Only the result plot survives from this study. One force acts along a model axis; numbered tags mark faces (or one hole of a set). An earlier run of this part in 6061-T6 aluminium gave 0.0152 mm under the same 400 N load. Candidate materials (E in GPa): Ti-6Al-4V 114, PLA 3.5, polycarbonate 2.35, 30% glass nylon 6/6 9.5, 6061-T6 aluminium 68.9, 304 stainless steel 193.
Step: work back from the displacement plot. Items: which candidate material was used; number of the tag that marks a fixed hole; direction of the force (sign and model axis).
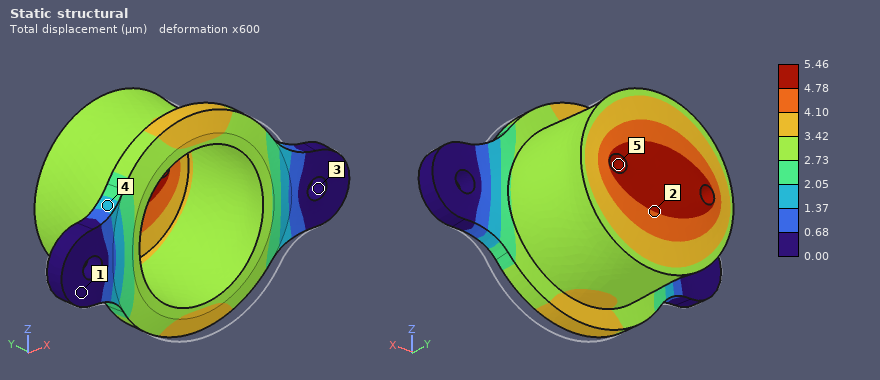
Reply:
304 stainless steel
3
+Y
